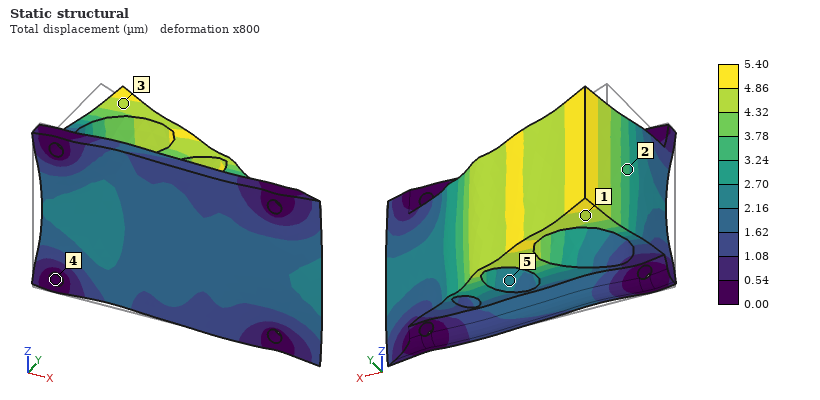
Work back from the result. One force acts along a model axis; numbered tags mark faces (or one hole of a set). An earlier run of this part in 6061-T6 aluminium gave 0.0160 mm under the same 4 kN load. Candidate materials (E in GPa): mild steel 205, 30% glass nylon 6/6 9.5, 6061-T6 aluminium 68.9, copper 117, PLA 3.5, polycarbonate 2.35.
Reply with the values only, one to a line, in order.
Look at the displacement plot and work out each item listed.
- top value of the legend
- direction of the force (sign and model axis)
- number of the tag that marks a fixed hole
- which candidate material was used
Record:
5.40 µm
+X
4
mild steel
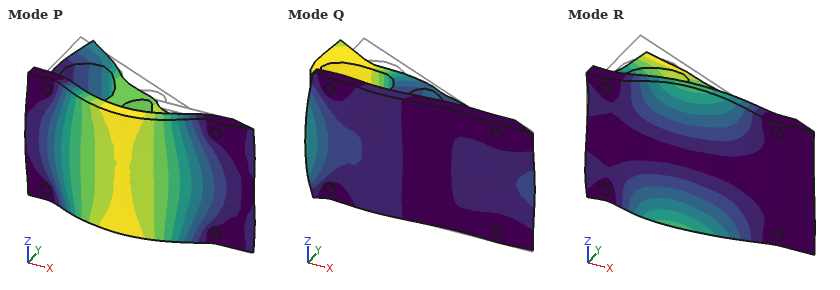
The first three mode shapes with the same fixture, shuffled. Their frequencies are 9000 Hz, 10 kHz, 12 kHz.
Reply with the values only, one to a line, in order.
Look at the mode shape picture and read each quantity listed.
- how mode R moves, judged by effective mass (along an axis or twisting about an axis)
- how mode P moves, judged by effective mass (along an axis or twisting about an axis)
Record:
along Z
along Y
